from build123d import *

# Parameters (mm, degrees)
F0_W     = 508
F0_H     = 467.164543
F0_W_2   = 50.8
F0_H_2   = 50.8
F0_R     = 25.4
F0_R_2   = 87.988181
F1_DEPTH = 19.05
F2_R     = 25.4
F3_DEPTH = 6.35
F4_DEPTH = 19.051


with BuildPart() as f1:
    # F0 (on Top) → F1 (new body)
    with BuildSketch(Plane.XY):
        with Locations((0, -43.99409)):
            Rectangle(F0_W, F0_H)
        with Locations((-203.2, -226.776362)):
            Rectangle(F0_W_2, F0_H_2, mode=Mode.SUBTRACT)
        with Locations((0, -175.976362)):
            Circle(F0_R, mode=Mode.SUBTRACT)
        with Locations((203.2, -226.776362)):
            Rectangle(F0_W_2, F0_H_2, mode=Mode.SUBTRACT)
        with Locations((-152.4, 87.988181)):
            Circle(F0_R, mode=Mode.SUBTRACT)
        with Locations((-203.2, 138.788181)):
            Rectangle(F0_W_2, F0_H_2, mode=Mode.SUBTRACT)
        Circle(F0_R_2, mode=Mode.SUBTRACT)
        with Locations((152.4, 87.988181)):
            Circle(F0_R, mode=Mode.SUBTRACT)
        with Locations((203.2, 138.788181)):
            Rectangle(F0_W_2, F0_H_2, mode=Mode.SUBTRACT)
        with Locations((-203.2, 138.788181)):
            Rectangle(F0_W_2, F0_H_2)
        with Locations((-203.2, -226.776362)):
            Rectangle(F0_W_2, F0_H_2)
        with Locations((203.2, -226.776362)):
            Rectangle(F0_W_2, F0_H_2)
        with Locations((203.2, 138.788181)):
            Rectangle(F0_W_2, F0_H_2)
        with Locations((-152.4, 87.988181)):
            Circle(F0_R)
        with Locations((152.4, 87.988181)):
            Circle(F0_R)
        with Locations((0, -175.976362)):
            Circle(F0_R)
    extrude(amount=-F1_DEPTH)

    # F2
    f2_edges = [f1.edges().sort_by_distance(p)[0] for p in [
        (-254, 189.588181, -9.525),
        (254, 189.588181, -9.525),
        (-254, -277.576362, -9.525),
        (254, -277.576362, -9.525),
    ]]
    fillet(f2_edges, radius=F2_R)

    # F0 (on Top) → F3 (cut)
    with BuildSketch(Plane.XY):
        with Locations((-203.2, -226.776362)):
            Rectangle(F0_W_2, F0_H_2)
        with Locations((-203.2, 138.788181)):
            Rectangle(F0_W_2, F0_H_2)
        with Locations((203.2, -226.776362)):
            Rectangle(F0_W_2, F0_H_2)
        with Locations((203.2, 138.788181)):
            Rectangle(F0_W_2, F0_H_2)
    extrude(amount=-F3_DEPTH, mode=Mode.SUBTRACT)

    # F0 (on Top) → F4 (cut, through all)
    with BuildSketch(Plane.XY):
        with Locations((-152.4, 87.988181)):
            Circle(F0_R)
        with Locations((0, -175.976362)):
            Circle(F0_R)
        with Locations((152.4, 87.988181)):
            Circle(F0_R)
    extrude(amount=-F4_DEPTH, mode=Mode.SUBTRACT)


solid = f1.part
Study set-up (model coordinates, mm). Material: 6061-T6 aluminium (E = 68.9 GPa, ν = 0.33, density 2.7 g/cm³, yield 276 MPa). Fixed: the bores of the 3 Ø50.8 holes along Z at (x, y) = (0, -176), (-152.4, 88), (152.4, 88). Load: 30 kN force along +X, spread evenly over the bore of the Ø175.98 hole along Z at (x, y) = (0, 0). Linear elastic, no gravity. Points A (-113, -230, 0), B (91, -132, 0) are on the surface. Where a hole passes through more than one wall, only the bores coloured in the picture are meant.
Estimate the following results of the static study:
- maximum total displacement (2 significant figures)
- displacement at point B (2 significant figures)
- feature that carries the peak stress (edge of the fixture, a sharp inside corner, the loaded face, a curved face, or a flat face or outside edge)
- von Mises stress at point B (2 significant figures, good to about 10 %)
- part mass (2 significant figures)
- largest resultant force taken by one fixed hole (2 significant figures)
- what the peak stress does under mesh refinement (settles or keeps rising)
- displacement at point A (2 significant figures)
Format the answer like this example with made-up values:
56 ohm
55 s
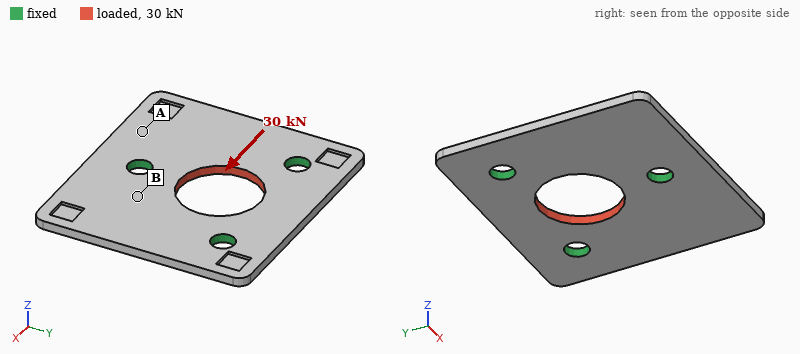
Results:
9.5 µm
4.8 µm
edge of the fixture
2.3 MPa
10 kg
11 kN
keeps rising
1.9 µm
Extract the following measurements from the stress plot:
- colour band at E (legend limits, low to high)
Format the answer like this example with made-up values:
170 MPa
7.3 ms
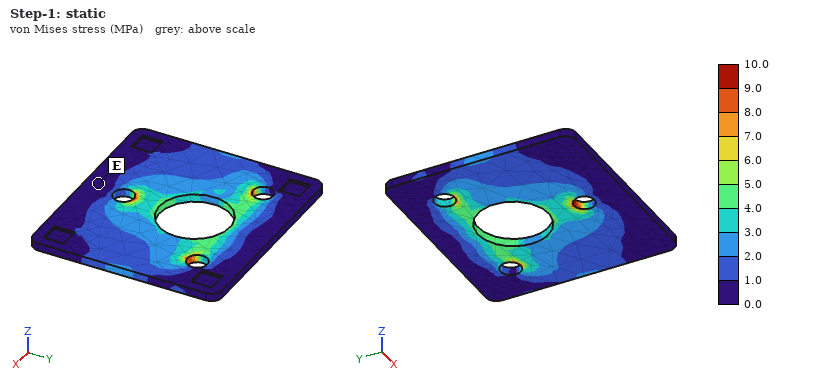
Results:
0.0 to 1.0 MPa
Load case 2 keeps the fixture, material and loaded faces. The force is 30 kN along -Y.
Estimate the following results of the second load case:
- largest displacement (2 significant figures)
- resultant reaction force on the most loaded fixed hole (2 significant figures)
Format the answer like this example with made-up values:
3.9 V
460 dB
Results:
15 µm
10 kN
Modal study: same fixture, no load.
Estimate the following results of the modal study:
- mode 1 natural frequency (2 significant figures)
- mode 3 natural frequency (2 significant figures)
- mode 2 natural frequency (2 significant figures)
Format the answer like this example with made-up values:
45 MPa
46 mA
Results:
370 Hz
920 Hz
380 Hz
